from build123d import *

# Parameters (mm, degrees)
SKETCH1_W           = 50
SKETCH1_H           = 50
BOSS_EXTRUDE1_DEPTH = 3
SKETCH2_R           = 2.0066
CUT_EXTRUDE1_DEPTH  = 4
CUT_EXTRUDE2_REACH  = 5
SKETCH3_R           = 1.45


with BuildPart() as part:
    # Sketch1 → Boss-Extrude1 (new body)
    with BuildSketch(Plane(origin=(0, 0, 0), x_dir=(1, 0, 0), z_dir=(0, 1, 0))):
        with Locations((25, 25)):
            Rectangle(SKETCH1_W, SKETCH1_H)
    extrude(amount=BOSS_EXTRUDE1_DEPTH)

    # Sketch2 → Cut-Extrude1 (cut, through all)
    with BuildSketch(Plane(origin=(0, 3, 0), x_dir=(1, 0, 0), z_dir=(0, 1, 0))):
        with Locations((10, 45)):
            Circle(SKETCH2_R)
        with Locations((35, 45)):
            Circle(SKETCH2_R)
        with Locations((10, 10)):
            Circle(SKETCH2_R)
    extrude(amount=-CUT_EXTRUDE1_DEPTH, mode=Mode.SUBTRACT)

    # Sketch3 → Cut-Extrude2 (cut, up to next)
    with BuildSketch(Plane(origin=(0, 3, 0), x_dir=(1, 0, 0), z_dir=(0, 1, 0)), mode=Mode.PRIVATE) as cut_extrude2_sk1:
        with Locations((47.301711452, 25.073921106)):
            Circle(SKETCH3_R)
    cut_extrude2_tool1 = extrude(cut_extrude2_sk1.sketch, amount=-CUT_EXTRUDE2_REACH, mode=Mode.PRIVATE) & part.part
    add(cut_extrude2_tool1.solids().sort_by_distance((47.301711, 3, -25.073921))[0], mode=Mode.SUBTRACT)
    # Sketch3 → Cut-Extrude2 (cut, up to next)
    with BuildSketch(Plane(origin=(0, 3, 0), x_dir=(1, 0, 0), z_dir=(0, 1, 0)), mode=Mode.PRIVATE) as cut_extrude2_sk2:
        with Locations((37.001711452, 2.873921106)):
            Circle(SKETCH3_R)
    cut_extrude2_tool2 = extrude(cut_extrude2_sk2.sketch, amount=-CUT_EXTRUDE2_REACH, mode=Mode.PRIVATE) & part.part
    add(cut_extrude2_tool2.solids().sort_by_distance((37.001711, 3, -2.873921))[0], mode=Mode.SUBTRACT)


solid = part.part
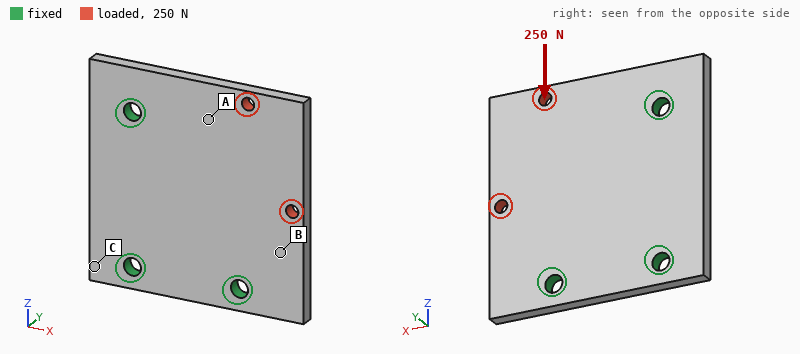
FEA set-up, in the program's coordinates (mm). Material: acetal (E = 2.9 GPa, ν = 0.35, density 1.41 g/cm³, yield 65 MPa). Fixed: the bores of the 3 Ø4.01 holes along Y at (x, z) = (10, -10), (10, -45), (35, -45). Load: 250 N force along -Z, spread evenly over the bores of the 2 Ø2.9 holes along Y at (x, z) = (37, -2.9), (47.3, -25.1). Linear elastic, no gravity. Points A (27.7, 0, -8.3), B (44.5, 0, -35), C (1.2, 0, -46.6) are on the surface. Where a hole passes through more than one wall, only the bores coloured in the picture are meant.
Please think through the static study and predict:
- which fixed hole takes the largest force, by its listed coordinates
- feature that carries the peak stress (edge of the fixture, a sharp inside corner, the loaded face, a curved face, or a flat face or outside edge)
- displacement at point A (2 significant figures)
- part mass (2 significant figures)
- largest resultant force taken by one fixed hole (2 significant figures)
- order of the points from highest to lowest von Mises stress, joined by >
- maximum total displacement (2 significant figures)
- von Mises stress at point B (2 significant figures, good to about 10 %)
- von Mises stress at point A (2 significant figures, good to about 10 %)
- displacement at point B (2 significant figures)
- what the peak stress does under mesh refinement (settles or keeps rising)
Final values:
(35, -45)
edge of the fixture
26 µm
10 g
190 N
B > A > C
63 µm
3.7 MPa
2.1 MPa
29 µm
keeps rising
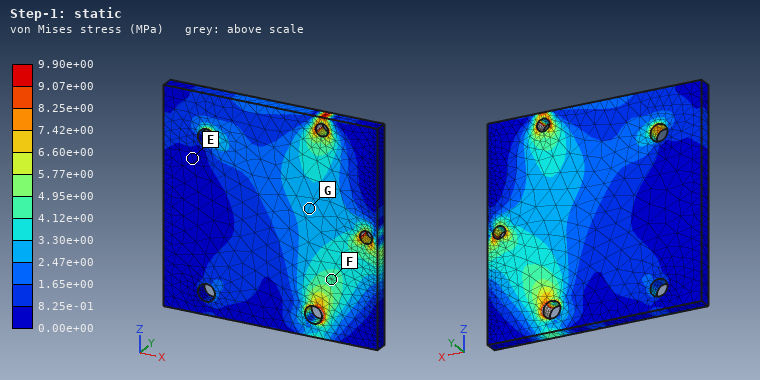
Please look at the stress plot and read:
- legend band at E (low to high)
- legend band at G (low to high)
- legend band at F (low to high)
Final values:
0.00e+00 to 8.25e-01 MPa
2.47e+00 to 3.30e+00 MPa
4.12e+00 to 4.95e+00 MPa
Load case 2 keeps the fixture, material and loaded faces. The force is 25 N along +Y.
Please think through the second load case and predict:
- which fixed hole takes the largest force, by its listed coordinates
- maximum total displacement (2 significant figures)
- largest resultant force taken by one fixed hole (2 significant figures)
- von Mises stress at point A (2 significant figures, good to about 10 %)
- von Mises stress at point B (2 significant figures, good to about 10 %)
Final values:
(35, -45)
0.80 mm
18 N
3.8 MPa
3.8 MPa
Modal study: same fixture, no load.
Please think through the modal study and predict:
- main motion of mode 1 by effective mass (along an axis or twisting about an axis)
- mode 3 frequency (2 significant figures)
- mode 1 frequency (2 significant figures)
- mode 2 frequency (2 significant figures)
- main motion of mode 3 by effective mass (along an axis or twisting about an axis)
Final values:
along Y
2800 Hz
740 Hz
2200 Hz
along Y
